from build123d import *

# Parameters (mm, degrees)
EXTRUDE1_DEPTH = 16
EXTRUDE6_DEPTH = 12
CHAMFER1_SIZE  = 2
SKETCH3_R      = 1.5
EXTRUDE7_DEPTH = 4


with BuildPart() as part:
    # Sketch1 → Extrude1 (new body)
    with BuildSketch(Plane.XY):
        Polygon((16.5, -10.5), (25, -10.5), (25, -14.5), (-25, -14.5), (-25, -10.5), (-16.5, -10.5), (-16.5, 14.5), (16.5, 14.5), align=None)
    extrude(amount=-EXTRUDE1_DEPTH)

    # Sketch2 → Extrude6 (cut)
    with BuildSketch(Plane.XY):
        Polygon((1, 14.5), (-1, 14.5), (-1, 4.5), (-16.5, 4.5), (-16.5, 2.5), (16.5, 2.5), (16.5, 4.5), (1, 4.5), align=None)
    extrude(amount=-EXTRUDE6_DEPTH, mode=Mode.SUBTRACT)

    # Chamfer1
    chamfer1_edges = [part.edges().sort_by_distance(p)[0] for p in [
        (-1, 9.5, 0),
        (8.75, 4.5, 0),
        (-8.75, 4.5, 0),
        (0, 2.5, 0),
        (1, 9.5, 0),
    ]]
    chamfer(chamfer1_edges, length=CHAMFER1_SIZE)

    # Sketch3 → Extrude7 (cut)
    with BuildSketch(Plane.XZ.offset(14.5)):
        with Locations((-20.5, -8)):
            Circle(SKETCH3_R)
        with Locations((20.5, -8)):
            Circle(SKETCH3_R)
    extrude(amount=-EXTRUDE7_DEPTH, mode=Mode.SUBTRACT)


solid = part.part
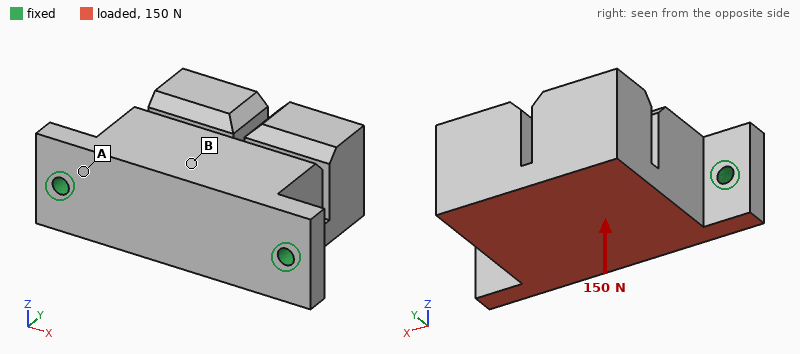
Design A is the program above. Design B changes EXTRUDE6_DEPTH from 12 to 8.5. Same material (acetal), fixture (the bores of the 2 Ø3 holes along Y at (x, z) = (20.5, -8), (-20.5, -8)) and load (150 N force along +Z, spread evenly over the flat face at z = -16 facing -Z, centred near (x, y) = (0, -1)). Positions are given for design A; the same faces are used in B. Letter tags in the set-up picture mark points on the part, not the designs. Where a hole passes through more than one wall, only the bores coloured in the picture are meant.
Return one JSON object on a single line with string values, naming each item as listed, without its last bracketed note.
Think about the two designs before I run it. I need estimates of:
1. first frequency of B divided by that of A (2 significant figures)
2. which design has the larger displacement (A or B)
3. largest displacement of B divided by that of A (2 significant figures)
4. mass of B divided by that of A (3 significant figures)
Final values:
{"first frequency of B divided by that of A": "1.0", "which design has the larger displacement": "A", "largest displacement of B divided by that of A": "0.91", "mass of B divided by that of A": "1.02"}
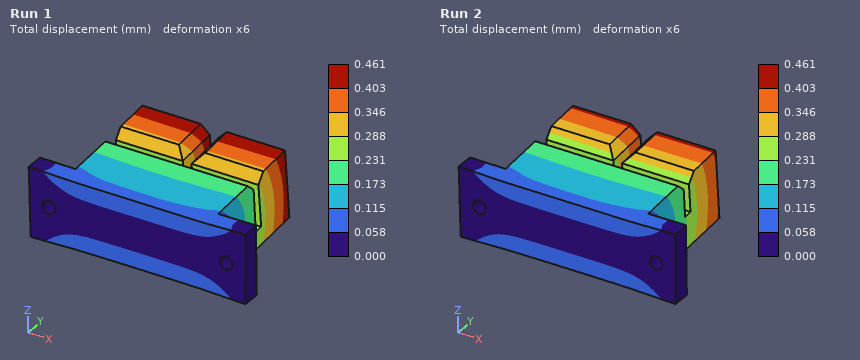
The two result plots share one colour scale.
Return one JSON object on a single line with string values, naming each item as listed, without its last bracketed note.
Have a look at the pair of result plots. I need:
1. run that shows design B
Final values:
{"run that shows design B": "Run 2"}
